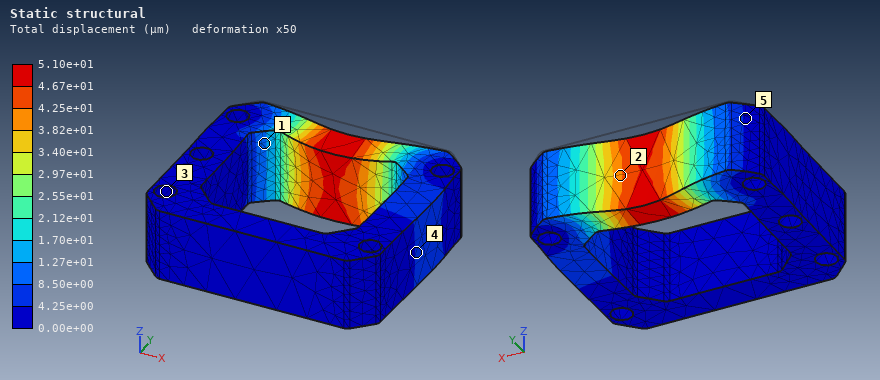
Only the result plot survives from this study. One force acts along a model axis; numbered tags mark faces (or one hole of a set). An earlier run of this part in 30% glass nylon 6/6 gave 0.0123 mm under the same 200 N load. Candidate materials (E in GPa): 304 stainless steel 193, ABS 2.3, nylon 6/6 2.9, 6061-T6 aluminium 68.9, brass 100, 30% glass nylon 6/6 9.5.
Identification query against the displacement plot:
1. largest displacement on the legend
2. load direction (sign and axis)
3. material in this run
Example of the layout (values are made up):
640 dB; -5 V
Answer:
5.10e+01 µm; -Y; ABS
